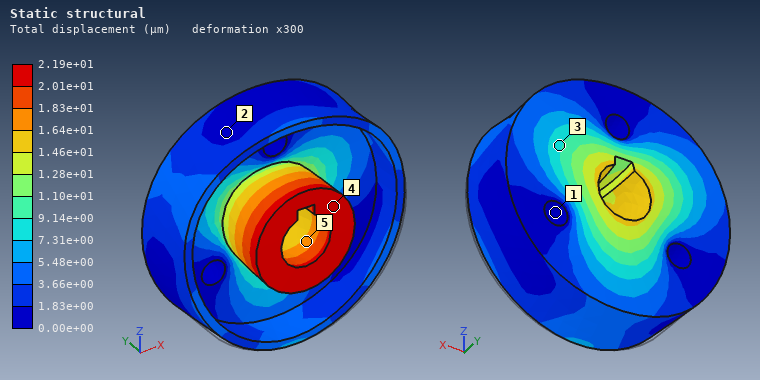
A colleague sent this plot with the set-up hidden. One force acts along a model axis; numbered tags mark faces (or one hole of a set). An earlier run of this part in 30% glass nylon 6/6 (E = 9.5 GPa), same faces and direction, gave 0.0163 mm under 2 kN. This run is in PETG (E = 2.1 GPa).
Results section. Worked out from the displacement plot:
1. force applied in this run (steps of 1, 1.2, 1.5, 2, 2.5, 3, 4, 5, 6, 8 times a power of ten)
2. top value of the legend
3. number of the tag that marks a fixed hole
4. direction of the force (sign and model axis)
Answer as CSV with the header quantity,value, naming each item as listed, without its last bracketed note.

quantity,value
force applied in this run,600 N
top value of the legend,2.19e+01 µm
number of the tag that marks a fixed hole,1
direction of the force,+Y
